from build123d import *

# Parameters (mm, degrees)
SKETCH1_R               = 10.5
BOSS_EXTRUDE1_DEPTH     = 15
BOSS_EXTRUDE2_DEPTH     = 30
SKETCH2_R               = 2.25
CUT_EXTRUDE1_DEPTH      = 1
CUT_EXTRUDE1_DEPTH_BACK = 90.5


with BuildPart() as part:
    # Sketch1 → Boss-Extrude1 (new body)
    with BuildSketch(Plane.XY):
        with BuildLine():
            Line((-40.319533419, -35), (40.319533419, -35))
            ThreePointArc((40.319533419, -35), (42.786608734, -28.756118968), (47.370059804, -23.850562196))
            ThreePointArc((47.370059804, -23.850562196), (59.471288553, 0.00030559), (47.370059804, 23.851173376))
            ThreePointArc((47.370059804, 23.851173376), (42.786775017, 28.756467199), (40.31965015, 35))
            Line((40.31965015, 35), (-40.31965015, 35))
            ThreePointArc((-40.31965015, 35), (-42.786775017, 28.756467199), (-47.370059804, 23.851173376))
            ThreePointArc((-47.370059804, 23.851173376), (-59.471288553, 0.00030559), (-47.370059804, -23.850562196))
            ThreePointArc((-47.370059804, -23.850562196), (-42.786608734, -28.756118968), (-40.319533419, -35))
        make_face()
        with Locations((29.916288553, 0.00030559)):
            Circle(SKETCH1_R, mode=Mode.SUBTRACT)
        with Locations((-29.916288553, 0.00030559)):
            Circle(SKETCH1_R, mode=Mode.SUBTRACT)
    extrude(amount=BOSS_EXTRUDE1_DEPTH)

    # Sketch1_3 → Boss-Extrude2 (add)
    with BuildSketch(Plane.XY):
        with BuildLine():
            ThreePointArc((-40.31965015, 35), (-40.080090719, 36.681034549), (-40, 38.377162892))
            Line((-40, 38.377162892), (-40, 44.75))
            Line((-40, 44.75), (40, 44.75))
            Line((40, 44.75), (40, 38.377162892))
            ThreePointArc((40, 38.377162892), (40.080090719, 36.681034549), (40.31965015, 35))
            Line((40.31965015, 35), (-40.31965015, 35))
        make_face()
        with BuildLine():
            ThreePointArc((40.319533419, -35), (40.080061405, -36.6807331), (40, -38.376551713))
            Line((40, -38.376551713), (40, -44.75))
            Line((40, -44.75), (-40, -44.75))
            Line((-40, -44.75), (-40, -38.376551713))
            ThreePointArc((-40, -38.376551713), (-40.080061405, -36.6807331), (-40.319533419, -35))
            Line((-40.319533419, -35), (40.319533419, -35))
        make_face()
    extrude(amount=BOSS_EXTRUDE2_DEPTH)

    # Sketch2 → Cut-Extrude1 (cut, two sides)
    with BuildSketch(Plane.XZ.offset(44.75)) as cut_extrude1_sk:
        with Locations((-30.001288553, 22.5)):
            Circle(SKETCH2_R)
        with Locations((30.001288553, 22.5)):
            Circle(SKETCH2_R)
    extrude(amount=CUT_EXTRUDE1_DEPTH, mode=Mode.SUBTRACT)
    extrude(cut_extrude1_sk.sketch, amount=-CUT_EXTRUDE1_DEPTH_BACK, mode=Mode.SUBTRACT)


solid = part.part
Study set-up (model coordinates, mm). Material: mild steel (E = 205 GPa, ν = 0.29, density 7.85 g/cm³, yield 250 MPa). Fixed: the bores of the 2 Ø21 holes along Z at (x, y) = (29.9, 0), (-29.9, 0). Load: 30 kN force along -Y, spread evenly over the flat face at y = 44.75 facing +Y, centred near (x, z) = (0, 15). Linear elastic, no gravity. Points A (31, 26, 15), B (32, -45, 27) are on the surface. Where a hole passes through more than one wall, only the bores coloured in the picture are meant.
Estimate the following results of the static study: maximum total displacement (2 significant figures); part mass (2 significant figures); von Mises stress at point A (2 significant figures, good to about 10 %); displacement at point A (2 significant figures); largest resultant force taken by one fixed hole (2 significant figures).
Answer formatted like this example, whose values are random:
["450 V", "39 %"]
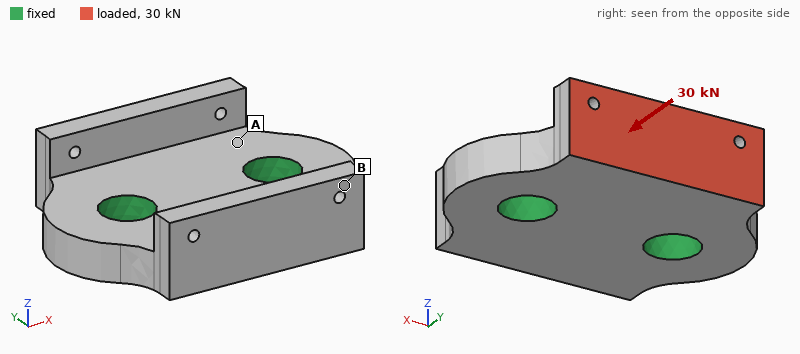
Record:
["60 µm", "1.1 kg", "89 MPa", "11 µm", "15 kN"]
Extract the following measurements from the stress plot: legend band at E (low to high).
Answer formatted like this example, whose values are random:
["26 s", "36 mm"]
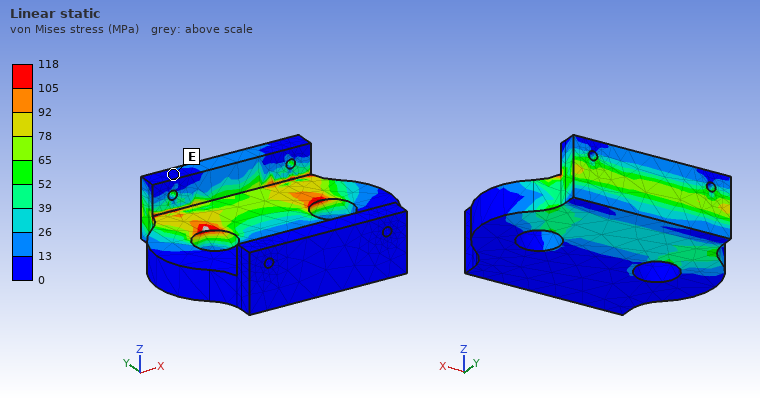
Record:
["0 to 13 MPa"]
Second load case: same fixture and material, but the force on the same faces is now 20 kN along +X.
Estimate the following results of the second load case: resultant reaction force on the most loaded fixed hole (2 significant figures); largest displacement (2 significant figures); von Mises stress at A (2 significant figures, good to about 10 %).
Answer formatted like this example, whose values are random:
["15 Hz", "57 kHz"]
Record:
["15 kN", "18 µm", "32 MPa"]
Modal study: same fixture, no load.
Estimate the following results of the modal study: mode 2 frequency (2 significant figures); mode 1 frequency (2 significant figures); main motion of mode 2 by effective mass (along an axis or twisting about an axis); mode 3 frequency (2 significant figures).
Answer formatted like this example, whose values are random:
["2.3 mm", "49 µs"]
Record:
["6000 Hz", "5700 Hz", "along Z", "9000 Hz"]
